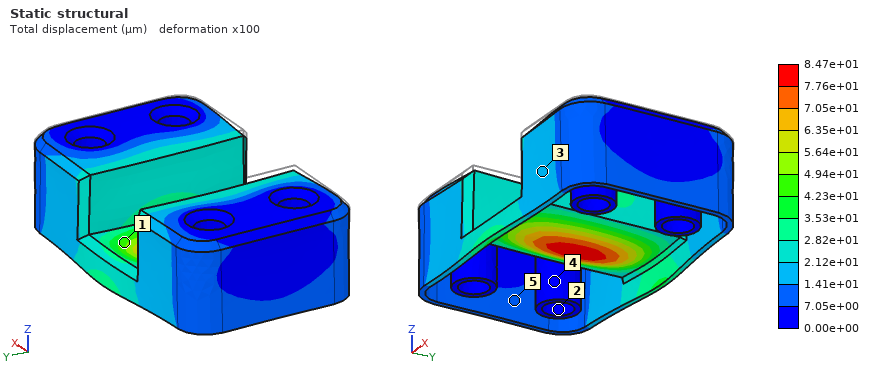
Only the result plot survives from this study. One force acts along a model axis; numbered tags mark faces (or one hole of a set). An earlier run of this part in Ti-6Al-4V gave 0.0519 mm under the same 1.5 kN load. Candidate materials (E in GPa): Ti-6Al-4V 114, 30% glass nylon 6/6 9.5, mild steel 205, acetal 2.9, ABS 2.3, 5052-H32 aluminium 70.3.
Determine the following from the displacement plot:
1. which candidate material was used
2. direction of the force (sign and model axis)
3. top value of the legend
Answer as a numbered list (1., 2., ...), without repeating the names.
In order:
1. 5052-H32 aluminium
2. -Z
3. 8.47e+01 µm
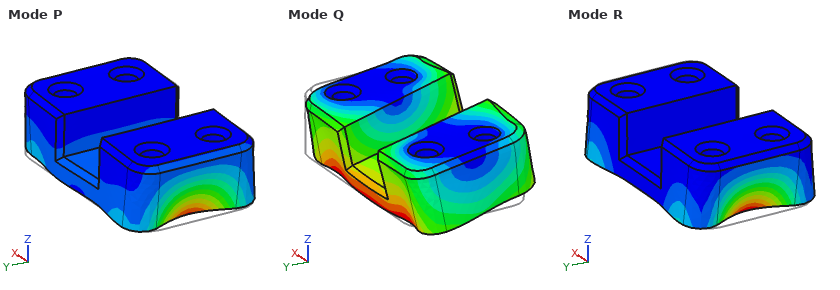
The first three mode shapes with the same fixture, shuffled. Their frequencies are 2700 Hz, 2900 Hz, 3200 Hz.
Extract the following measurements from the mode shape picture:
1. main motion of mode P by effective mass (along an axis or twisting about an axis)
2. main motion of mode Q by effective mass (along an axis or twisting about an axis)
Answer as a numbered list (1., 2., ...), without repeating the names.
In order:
1. along X
2. along Y
